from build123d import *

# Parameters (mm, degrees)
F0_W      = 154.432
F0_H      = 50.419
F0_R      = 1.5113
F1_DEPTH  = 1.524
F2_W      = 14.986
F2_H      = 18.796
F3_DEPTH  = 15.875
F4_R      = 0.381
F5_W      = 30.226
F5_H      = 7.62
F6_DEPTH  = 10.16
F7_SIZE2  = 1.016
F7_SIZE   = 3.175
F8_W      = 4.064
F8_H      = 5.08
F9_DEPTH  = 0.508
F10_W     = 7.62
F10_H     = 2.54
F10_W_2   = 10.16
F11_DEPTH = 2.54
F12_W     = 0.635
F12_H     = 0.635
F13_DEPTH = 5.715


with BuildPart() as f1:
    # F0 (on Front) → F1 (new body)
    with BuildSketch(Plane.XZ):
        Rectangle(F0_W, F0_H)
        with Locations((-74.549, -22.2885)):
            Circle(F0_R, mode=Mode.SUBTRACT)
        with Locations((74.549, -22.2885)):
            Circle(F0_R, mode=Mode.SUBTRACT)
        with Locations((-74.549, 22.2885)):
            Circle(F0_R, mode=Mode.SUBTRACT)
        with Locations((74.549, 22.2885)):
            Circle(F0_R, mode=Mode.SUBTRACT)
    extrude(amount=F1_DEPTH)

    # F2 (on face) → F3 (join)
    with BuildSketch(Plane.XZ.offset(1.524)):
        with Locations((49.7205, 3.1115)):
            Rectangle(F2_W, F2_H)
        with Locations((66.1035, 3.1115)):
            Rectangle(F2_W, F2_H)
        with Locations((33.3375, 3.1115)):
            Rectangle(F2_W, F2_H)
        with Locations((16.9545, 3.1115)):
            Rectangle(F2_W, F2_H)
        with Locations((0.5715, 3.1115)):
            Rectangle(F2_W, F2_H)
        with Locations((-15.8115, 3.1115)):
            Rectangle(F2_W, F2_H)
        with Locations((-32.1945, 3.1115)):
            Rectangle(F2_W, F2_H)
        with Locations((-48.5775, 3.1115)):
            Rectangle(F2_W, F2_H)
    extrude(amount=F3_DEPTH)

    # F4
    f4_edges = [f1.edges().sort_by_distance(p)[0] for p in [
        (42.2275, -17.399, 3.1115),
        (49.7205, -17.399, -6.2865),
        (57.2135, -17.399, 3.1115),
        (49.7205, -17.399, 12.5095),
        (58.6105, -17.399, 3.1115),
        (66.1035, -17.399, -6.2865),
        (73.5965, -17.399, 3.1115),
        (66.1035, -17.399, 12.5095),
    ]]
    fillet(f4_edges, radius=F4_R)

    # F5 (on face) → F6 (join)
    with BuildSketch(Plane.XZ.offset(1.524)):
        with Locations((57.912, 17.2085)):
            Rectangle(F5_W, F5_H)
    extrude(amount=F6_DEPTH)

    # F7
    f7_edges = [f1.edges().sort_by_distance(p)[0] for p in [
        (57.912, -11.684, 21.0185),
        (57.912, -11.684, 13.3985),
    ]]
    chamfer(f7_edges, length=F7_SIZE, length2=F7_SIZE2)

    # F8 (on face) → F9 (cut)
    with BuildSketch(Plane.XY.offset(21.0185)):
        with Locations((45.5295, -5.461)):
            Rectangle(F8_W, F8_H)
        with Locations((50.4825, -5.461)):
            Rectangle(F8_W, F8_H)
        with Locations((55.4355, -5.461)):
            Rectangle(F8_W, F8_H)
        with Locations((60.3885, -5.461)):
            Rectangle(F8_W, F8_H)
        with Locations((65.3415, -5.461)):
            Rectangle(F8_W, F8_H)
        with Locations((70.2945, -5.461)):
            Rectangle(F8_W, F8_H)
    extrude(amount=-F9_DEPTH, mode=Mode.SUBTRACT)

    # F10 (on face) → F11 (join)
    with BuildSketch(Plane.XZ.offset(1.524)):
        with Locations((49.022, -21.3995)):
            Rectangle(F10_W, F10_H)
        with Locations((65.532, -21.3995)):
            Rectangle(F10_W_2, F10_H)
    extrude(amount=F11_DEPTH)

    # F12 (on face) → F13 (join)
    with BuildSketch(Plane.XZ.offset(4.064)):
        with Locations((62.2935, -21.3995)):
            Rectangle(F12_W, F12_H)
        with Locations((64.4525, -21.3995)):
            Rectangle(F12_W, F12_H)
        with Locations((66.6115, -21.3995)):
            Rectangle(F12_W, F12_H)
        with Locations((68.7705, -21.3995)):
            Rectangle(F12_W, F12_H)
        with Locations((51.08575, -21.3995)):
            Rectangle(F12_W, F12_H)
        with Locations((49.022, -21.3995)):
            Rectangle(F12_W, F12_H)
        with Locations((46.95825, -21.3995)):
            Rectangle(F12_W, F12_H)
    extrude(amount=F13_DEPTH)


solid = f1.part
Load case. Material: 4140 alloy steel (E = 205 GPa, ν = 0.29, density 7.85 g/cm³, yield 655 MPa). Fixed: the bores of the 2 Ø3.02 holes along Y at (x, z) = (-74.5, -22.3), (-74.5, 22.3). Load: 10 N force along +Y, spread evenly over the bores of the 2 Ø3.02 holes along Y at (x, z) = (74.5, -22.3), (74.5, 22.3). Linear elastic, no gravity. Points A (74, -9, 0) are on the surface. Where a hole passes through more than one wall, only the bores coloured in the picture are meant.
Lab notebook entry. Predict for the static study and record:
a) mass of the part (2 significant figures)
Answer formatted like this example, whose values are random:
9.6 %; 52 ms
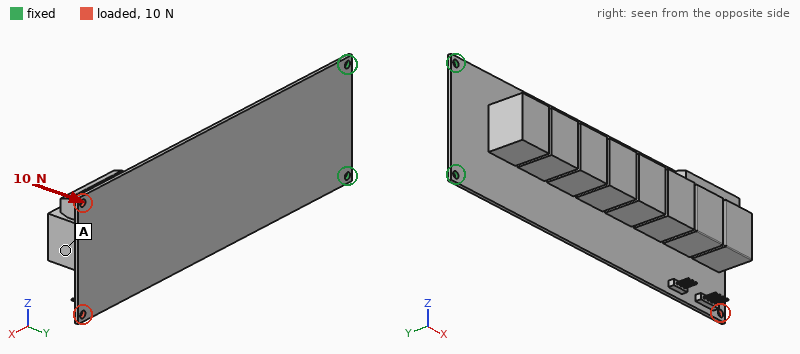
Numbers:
390 g
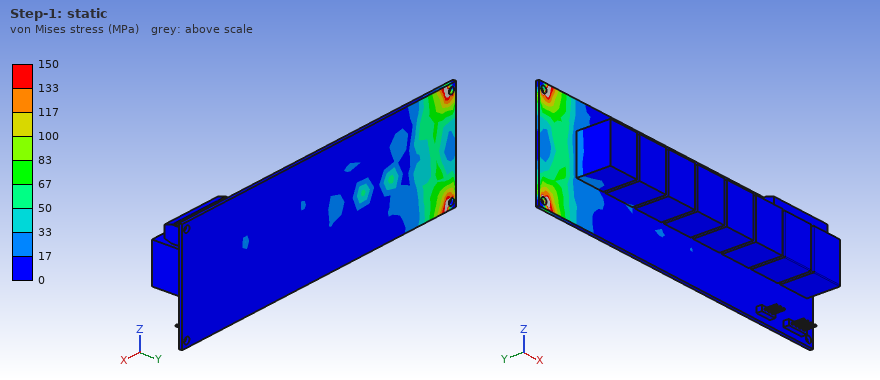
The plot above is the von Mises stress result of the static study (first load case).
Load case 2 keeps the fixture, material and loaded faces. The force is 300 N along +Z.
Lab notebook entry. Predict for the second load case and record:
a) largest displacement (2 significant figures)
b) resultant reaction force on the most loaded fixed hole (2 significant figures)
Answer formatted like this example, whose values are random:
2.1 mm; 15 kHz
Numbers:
0.12 mm; 1.0 kN
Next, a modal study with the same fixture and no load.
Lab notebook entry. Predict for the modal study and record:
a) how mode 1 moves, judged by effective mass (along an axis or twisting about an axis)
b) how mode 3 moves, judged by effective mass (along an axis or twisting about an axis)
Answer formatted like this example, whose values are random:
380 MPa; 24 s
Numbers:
along Y; along Z
